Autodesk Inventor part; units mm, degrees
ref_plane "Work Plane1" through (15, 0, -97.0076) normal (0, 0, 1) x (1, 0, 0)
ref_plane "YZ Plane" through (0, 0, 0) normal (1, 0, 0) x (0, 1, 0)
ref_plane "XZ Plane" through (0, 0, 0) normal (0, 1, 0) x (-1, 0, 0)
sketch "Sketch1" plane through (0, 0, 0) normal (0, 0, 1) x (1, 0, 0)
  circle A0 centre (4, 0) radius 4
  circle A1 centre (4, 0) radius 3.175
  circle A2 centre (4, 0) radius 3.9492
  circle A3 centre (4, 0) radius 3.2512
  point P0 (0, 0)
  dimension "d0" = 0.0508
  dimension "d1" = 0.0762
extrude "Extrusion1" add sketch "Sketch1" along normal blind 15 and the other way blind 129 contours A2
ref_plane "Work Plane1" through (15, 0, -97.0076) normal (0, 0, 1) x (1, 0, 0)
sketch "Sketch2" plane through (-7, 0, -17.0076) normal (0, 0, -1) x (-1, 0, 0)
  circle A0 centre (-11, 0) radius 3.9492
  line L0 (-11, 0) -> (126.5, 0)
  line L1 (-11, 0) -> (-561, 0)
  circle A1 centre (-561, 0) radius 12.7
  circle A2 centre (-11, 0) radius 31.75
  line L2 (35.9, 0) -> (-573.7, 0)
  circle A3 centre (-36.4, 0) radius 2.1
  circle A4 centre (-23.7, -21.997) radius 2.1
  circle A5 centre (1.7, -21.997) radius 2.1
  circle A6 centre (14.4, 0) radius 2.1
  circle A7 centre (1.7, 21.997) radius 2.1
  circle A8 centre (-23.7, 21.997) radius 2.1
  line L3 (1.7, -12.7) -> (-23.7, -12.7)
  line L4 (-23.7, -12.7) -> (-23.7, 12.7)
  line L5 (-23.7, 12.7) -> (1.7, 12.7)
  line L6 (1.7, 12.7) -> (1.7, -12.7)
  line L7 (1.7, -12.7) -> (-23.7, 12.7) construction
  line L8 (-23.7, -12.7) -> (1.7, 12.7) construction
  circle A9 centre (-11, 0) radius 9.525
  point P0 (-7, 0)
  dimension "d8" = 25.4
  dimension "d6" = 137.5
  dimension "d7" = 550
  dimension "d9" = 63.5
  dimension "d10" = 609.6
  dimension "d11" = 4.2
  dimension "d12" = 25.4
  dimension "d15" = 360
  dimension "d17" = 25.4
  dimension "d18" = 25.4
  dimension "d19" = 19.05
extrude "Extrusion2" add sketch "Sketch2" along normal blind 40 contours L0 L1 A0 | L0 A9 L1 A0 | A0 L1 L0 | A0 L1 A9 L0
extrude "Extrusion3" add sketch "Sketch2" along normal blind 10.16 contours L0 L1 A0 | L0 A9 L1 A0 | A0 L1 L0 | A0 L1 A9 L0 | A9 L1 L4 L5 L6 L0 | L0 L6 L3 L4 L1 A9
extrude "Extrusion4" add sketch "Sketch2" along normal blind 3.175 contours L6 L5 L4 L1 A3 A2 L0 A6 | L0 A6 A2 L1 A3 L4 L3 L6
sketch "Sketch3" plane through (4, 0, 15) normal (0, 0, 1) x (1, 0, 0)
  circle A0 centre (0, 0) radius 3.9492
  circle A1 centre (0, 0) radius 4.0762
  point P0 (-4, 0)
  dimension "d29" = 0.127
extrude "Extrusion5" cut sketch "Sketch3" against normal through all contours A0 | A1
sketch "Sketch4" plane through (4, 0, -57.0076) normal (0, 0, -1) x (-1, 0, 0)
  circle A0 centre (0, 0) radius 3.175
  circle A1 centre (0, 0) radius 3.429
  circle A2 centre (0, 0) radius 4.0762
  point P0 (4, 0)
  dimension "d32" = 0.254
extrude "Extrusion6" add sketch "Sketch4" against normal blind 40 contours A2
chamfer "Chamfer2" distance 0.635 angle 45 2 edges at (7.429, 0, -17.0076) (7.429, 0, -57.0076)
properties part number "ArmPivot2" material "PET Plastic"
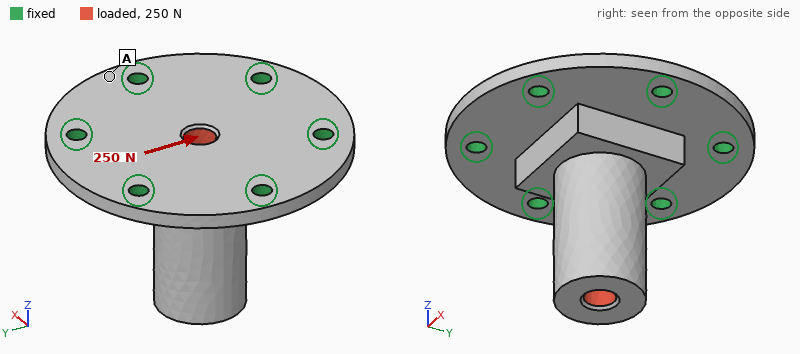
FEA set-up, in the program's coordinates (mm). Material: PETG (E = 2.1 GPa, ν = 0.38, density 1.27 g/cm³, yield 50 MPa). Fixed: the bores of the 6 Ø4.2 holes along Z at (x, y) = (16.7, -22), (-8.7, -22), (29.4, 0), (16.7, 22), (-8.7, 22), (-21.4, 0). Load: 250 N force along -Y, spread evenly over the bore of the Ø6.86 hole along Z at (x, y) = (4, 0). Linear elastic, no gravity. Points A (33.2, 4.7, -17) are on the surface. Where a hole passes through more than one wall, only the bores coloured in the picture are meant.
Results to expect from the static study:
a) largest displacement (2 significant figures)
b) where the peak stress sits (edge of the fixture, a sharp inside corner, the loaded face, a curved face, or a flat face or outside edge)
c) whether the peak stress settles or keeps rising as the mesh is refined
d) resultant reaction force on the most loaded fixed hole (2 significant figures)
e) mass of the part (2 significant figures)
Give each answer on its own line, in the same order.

0.34 mm
edge of the fixture
keeps rising
88 N
27 g
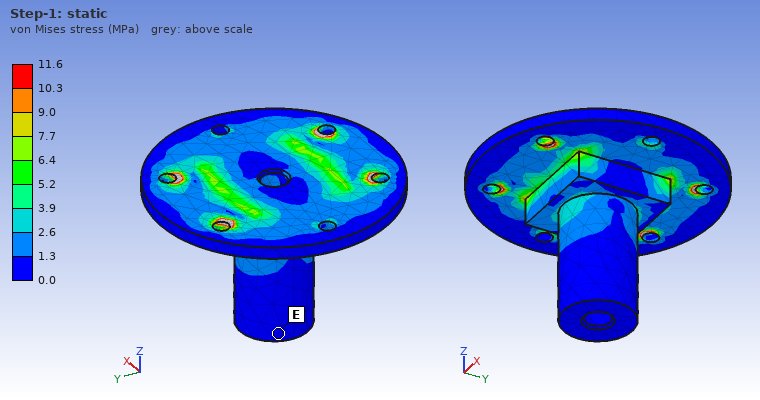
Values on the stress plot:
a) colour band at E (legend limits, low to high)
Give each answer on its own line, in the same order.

0.0 to 1.3 MPa
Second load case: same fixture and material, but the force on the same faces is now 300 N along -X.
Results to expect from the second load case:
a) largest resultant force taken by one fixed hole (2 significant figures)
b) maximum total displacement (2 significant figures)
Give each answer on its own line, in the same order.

100 N
0.42 mm
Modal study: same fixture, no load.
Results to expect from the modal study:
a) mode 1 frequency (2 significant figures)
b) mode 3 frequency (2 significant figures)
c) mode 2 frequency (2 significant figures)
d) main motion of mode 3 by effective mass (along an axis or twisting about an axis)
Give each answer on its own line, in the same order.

1400 Hz
2100 Hz
1400 Hz
along Z
